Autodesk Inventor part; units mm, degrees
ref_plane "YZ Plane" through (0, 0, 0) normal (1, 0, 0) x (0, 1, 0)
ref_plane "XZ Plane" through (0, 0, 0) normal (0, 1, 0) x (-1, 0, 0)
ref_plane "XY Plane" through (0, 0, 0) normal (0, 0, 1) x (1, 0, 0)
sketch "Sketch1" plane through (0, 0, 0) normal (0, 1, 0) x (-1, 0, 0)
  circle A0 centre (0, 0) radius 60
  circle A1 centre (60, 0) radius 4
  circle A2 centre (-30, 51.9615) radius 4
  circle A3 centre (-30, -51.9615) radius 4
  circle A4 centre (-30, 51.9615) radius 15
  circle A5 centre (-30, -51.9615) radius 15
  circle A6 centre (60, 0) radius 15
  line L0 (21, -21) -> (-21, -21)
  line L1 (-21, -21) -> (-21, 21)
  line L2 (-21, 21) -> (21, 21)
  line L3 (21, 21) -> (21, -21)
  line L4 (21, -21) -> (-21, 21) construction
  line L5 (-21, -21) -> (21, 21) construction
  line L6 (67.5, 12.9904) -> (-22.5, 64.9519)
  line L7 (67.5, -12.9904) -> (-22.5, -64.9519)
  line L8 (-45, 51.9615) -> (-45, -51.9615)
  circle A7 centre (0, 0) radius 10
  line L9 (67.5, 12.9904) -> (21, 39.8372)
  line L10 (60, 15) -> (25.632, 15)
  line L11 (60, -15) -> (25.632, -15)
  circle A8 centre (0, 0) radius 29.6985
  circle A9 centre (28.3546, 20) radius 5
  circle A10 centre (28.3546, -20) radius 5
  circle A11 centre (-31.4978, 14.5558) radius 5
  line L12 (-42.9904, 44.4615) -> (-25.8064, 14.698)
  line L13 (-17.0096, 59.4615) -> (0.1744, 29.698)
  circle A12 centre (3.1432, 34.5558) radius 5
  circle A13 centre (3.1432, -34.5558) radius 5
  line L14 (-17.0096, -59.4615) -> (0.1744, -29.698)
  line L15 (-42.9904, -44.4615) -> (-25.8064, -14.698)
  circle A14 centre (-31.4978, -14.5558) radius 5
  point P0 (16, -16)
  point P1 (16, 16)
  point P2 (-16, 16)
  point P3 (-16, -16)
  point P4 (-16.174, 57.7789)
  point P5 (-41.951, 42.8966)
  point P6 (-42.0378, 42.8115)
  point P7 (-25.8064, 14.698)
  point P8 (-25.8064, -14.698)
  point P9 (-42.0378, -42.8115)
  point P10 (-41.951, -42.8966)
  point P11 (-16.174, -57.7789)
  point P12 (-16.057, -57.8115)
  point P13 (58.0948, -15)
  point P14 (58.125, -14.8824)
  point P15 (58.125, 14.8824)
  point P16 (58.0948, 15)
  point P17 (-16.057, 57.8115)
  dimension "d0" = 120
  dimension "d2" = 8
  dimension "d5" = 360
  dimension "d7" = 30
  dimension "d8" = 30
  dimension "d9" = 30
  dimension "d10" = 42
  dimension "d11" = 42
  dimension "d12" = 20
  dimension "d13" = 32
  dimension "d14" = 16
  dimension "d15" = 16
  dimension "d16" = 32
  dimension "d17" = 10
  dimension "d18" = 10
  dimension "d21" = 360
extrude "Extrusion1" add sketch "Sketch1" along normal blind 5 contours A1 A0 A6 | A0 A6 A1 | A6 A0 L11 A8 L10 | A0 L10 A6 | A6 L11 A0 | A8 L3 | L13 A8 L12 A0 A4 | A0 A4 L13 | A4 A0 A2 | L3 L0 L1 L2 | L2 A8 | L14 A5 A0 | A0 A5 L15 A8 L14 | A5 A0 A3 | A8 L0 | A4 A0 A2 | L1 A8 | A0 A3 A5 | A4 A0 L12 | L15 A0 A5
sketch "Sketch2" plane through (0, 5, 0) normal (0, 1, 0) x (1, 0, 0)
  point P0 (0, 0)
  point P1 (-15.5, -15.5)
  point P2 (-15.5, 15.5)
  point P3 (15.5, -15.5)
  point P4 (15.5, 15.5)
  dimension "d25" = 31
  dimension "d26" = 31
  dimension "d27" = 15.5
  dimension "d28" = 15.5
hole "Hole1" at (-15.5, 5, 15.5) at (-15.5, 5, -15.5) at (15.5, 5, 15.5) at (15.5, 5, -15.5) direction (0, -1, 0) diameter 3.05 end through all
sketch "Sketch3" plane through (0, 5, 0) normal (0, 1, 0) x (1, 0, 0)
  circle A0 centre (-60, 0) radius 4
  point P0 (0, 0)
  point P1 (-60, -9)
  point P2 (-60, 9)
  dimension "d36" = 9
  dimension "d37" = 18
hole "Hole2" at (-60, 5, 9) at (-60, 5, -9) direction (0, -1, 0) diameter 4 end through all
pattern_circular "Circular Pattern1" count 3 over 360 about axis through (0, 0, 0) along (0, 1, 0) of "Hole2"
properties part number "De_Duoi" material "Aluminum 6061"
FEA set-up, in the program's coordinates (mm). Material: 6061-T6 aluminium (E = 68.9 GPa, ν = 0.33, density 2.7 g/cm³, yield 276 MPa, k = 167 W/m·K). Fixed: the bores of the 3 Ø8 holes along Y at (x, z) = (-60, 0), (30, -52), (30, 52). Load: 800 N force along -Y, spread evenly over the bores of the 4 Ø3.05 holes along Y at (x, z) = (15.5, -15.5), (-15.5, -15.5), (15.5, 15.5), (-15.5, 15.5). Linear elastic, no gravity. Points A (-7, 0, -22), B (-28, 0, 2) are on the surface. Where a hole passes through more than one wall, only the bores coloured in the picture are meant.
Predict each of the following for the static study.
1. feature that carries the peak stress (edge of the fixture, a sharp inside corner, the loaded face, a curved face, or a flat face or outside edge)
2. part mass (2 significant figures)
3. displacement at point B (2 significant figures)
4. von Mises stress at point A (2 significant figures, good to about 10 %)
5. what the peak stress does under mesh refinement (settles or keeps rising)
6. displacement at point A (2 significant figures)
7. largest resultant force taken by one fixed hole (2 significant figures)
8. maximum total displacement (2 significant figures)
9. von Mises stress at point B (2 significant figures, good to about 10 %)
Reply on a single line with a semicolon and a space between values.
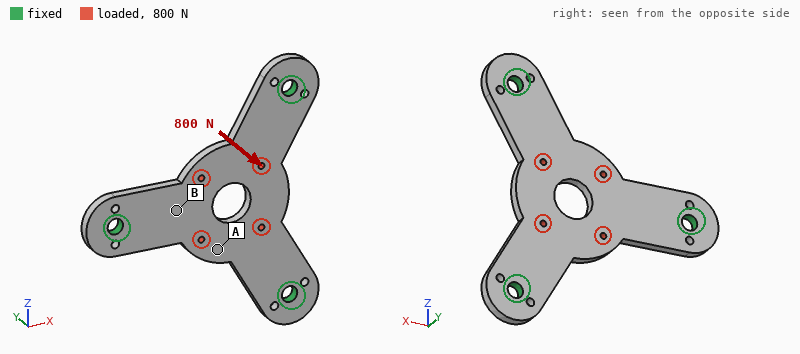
edge of the fixture; 82 g; 0.082 mm; 25 MPa; keeps rising; 0.11 mm; 270 N; 0.13 mm; 10 MPa
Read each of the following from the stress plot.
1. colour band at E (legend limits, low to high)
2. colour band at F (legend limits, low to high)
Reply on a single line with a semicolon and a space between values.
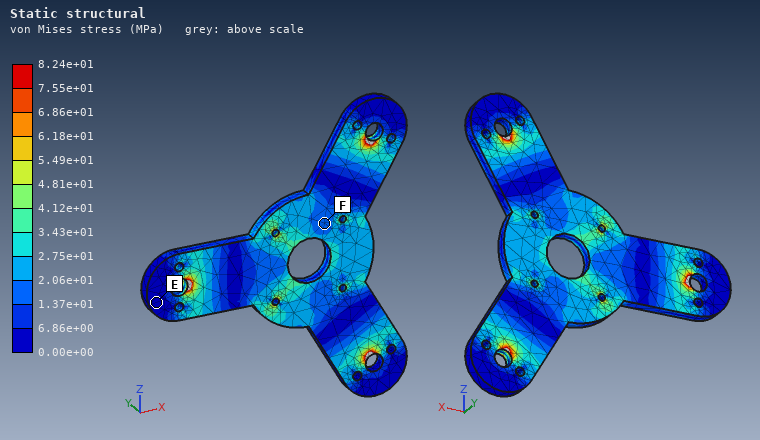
0.00e+00 to 6.86e+00 MPa; 1.37e+01 to 2.06e+01 MPa
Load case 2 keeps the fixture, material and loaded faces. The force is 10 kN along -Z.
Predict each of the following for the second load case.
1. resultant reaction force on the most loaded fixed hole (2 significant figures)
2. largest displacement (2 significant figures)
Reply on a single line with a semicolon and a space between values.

4.9 kN; 52 µm
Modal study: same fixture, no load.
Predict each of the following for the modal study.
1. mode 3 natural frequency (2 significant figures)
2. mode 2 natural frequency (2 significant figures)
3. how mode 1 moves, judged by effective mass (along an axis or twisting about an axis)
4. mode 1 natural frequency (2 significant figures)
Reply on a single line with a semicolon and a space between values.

4200 Hz; 4200 Hz; along Y; 2200 Hz
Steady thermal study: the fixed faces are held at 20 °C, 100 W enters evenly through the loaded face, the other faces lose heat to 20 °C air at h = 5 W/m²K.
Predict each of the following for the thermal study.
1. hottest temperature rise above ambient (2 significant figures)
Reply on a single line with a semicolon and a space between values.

63 K
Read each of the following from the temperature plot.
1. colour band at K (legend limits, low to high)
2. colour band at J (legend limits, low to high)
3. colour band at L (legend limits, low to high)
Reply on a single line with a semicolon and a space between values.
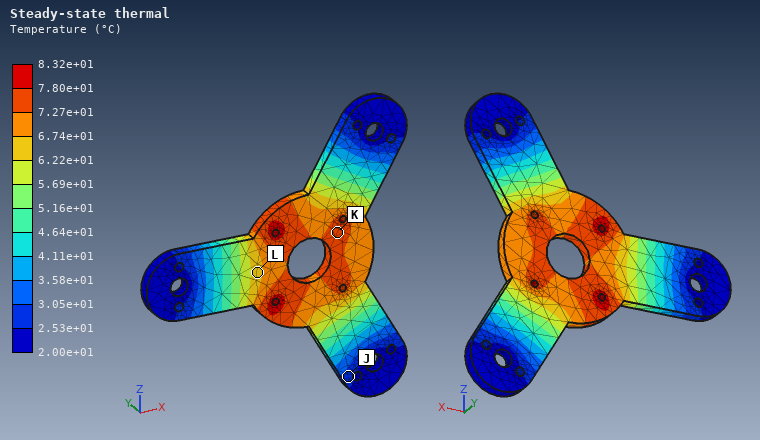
7.27e+01 to 7.80e+01 °C; 2.53e+01 to 3.05e+01 °C; 6.22e+01 to 6.74e+01 °C
